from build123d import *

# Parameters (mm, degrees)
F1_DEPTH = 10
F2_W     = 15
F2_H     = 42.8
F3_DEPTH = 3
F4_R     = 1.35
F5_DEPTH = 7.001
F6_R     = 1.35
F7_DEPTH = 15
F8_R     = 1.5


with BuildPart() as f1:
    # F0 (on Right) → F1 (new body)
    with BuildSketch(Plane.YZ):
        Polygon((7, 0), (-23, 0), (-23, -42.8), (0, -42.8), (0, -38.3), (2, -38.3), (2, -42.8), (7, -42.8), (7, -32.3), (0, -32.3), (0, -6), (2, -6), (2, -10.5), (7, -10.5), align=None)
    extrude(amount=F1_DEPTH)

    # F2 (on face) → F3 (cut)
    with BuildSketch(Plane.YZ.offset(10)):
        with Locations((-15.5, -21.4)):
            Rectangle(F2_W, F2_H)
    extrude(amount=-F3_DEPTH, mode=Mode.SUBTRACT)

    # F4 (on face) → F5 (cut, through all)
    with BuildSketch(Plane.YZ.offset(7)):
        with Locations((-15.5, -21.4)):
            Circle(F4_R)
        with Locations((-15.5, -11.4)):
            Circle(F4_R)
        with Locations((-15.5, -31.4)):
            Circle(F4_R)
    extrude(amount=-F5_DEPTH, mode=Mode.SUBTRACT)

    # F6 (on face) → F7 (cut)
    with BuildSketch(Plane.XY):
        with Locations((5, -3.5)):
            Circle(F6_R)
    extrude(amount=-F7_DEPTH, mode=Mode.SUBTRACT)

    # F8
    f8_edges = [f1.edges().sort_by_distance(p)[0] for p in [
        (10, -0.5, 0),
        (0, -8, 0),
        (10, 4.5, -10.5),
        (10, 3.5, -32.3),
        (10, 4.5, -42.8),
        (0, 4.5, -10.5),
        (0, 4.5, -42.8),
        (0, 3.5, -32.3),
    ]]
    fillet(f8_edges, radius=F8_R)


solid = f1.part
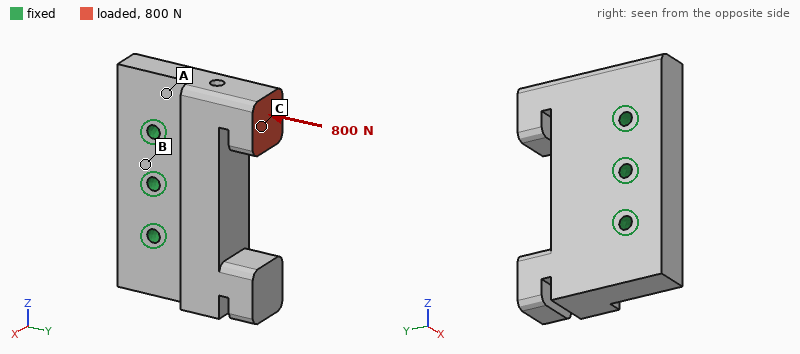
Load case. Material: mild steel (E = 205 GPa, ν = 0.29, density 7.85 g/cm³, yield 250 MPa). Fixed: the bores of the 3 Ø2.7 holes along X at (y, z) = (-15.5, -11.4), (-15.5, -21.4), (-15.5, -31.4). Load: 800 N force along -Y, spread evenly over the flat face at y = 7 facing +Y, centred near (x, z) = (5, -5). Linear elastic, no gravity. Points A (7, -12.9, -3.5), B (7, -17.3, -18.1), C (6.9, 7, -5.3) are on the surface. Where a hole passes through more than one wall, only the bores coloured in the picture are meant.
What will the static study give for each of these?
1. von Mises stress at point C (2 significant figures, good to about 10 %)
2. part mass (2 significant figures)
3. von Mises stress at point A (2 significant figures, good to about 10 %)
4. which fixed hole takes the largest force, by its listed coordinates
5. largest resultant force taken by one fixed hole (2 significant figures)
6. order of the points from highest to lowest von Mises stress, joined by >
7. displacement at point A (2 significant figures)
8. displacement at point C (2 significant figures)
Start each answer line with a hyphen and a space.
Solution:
- 19 MPa
- 70 g
- 11 MPa
- (-15.5, -11.4)
- 980 N
- C > A > B
- 1.2 µm
- 3.5 µm
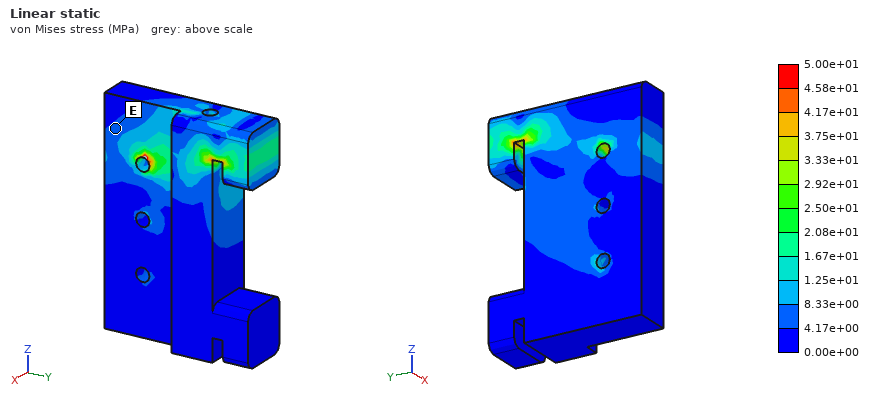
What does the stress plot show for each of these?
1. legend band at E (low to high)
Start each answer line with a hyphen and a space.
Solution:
- 4.17e+00 to 8.33e+00 MPa
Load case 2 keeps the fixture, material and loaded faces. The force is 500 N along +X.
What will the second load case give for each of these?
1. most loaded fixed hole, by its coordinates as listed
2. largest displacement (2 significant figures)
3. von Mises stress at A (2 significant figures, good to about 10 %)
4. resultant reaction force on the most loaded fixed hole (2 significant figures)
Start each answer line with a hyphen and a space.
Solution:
- (-15.5, -11.4)
- 22 µm
- 34 MPa
- 470 N
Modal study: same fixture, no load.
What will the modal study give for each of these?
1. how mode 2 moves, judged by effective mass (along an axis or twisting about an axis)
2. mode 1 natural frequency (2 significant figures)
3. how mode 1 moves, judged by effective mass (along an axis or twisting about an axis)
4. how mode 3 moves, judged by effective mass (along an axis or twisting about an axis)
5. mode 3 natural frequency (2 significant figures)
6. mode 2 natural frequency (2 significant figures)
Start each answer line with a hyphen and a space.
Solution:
- twisting about Y
- 10 kHz
- along X
- along Z
- 18 kHz
- 12 kHz
